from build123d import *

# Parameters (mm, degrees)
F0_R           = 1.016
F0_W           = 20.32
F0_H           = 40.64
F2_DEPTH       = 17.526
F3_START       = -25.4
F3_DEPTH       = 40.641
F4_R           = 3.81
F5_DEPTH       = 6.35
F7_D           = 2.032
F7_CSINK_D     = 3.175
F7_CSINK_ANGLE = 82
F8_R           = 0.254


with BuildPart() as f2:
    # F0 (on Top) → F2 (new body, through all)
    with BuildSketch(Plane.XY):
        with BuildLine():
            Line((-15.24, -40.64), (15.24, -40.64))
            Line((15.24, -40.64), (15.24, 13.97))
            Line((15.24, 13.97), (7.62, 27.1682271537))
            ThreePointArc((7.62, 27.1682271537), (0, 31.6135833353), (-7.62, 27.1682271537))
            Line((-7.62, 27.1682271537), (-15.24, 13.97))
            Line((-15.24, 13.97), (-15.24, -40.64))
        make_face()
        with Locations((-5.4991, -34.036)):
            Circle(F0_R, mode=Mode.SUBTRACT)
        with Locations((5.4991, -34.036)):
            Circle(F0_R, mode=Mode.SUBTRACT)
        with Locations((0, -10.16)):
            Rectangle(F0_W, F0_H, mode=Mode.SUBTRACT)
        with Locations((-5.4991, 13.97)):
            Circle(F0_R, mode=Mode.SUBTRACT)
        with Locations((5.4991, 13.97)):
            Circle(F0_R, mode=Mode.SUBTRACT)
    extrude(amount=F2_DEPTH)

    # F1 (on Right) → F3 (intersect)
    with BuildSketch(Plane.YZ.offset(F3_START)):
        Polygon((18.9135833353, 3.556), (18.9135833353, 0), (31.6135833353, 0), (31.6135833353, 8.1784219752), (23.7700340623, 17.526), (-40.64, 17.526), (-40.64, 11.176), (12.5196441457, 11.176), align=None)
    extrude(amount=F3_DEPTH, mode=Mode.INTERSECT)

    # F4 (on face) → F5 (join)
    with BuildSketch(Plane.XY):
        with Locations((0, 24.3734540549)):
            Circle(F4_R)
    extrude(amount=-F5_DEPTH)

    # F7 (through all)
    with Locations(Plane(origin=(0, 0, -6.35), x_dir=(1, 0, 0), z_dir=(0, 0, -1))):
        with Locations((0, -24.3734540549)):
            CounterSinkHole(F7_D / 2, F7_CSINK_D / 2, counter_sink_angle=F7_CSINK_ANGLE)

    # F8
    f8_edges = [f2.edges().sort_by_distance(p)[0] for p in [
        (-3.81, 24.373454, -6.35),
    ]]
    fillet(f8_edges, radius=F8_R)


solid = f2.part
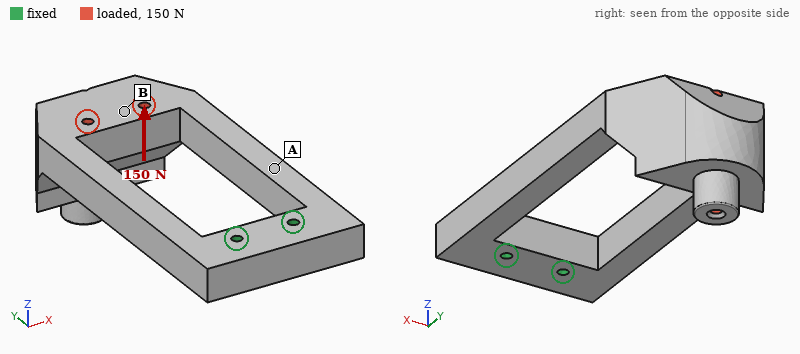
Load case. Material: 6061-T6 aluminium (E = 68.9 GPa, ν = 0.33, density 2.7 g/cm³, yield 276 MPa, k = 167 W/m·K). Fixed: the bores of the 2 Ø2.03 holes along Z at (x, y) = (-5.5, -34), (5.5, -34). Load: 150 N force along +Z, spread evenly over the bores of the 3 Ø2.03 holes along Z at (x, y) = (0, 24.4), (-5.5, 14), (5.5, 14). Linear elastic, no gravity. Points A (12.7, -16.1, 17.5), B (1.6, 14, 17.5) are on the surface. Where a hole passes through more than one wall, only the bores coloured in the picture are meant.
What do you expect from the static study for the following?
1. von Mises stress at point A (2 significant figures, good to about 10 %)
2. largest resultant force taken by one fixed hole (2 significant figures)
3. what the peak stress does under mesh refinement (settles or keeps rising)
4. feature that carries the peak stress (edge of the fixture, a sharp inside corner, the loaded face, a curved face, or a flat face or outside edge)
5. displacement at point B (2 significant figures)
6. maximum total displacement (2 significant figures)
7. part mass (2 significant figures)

79 MPa
75 N
keeps rising
edge of the fixture
0.53 mm
0.85 mm
28 g
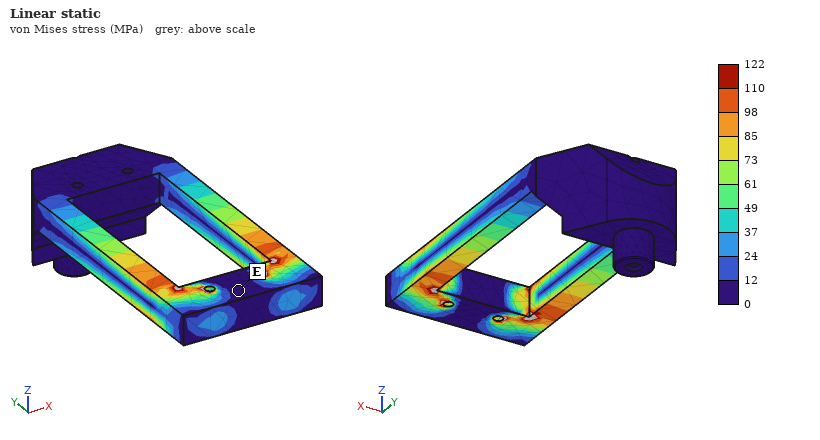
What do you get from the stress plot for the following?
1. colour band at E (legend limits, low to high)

0 to 12 MPa
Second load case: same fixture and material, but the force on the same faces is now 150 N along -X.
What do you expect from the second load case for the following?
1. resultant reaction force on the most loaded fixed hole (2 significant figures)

580 N
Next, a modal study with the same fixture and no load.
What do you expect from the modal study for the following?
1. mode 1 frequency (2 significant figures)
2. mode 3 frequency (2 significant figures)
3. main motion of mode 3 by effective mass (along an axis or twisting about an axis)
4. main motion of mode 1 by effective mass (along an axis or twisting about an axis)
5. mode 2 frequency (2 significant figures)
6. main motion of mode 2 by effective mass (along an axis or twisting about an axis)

580 Hz
2400 Hz
twisting about Y
along Z
1100 Hz
along X
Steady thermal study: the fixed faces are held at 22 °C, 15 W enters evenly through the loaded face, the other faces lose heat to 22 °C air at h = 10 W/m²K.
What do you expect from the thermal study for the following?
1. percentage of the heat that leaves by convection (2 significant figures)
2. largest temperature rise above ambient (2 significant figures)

13 %
67 K
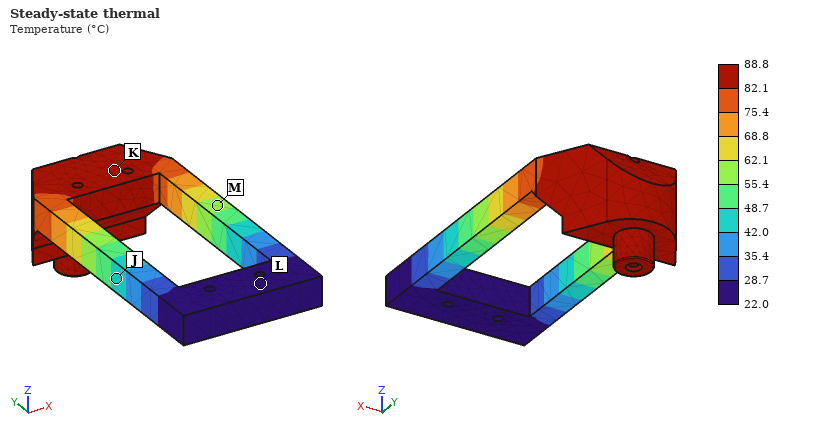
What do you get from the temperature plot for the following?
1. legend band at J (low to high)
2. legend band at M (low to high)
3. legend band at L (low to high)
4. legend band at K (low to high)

42.0 to 48.7 °C
55.4 to 62.1 °C
22.0 to 28.7 °C
82.1 to 88.8 °C
